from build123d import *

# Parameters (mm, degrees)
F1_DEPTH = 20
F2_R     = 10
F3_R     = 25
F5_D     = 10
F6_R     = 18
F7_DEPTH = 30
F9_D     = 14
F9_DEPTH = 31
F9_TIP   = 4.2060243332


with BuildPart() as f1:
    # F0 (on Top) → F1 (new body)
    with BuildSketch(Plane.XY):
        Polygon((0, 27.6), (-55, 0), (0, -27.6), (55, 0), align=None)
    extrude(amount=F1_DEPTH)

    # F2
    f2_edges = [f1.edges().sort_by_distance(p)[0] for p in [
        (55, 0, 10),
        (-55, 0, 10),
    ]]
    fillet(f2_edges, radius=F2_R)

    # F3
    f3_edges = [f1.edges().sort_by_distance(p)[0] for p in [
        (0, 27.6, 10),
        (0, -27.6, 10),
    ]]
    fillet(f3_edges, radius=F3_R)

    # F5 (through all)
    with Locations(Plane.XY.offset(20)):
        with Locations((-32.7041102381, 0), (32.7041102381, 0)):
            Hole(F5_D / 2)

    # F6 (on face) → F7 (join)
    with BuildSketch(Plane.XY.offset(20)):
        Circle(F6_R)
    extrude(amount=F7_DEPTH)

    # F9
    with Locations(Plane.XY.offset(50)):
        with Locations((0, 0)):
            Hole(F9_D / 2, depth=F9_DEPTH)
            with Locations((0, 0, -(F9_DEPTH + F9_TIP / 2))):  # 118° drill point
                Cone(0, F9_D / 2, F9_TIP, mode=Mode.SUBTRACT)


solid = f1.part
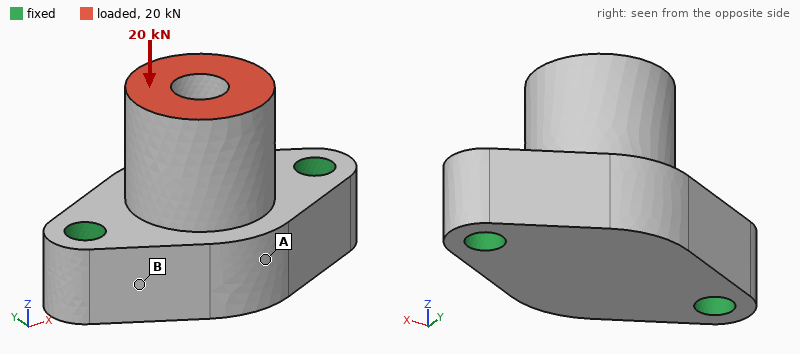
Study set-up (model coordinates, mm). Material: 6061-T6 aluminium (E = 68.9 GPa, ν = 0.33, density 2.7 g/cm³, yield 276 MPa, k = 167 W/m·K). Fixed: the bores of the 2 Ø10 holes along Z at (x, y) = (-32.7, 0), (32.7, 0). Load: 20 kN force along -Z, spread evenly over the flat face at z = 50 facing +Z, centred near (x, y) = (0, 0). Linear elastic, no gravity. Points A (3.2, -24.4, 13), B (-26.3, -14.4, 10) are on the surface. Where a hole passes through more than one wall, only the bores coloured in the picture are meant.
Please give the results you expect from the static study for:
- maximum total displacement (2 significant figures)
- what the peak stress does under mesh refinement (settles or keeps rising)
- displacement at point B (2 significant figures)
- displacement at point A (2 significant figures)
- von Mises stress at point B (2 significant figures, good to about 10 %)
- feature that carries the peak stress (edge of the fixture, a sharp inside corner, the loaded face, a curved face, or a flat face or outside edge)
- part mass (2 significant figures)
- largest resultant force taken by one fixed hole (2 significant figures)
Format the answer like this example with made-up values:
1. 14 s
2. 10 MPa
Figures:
1. 31 µm
2. keeps rising
3. 7.4 µm
4. 24 µm
5. 30 MPa
6. edge of the fixture
7. 210 g
8. 10 kN
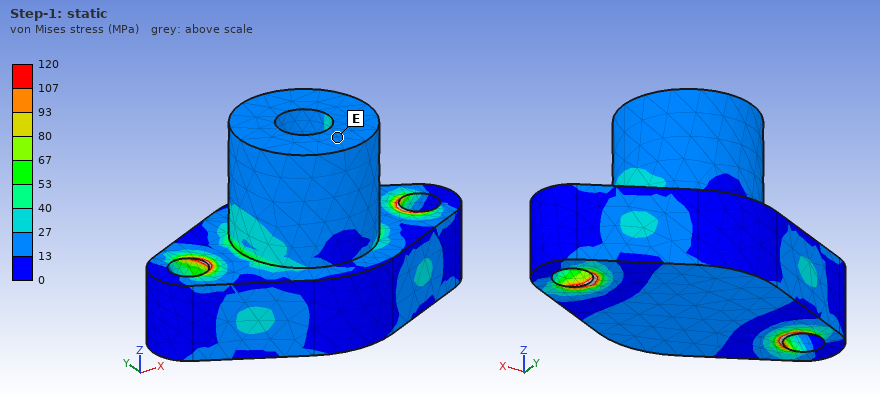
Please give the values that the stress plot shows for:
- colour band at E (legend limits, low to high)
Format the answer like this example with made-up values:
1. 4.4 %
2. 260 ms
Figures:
1. 13 to 27 MPa
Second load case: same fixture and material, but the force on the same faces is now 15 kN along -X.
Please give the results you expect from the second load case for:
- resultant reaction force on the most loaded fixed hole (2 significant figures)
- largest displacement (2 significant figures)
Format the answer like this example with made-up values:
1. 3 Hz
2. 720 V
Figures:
1. 13 kN
2. 0.11 mm
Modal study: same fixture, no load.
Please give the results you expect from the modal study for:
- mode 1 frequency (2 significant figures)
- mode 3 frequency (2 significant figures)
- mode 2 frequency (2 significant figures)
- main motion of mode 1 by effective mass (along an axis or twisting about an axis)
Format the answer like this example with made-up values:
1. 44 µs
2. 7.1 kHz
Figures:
1. 6300 Hz
2. 12 kHz
3. 12 kHz
4. along Y
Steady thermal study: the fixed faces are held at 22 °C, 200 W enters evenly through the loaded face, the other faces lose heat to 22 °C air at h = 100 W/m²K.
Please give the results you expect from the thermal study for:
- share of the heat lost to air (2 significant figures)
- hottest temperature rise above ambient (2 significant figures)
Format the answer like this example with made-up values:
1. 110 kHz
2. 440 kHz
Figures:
1. 14 %
2. 61 K
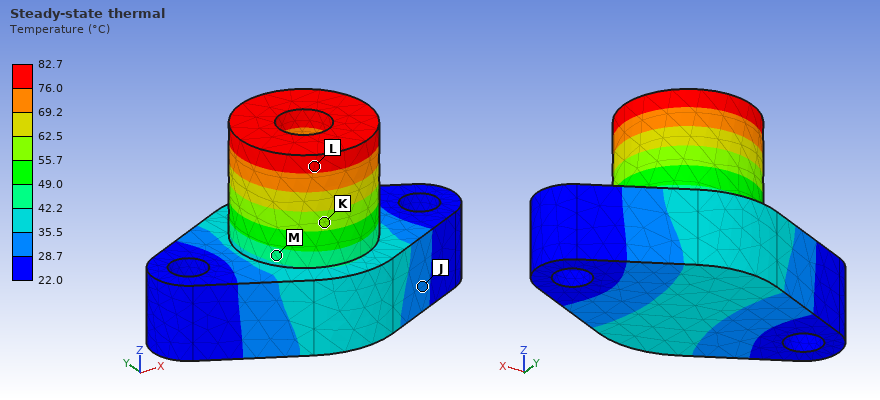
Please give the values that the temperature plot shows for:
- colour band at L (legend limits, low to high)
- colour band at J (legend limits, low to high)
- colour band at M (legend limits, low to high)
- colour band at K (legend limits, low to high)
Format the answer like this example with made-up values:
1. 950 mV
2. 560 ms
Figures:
1. 76.0 to 82.7 °C
2. 28.7 to 35.5 °C
3. 42.2 to 49.0 °C
4. 55.7 to 62.5 °C
